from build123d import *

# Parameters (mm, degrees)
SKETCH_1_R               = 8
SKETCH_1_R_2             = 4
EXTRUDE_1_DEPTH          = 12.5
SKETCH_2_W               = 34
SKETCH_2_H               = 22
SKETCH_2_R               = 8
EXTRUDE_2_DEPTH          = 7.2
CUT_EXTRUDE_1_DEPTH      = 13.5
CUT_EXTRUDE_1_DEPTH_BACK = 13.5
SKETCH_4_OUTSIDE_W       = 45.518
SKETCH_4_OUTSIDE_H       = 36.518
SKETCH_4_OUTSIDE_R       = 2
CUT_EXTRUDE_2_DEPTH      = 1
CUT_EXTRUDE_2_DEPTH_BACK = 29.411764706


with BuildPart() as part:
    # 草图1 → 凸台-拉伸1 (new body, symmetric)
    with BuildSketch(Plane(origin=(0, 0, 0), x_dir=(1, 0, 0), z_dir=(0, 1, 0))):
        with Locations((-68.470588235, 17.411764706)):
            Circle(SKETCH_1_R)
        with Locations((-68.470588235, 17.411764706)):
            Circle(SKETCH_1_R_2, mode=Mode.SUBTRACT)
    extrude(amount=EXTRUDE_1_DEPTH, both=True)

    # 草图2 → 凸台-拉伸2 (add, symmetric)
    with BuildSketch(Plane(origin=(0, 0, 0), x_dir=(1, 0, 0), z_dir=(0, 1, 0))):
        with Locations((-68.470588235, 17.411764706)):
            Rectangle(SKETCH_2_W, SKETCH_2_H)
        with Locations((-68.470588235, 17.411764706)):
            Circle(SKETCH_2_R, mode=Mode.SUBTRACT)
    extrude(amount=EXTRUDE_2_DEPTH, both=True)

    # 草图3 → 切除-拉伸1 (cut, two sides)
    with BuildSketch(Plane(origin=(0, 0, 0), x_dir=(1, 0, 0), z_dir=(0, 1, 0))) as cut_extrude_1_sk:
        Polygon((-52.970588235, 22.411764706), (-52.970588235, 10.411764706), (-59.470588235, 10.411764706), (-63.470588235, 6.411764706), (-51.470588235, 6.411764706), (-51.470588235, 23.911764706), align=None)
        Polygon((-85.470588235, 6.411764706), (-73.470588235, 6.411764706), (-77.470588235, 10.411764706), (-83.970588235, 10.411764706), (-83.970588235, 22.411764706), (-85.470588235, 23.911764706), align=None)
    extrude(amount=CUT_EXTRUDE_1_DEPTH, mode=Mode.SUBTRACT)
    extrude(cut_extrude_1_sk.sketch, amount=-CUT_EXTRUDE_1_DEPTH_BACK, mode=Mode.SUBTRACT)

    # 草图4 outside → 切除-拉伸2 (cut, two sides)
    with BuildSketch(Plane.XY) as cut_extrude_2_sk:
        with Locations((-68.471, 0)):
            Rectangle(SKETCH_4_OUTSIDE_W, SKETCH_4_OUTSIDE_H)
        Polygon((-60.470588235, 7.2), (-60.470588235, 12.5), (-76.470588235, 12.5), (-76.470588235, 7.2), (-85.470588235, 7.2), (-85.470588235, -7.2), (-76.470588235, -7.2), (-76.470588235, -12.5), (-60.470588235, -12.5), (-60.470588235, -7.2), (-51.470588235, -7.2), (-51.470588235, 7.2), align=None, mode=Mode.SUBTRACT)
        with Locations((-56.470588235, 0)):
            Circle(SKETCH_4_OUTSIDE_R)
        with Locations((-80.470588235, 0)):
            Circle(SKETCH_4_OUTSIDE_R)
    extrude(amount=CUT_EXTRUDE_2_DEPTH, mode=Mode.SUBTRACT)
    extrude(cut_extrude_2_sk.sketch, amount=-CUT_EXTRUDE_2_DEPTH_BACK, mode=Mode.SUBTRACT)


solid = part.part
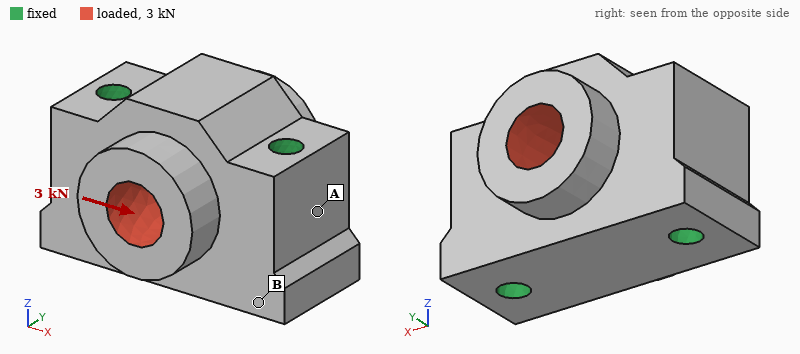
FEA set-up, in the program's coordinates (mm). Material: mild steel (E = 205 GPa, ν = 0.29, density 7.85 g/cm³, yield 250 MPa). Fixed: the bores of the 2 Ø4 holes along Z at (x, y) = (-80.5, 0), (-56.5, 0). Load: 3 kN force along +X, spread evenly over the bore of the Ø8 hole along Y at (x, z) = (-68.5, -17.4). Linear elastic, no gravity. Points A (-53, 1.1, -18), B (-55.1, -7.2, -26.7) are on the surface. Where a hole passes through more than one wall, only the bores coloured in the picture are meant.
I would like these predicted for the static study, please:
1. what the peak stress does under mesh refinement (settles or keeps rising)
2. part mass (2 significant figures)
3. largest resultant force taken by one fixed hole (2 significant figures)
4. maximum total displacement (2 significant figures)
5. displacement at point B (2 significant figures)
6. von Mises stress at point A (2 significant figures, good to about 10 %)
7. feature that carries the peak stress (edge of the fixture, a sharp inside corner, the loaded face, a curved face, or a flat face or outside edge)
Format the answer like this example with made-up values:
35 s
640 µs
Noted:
keeps rising
75 g
1.5 kN
0.82 µm
0.14 µm
5.3 MPa
edge of the fixture
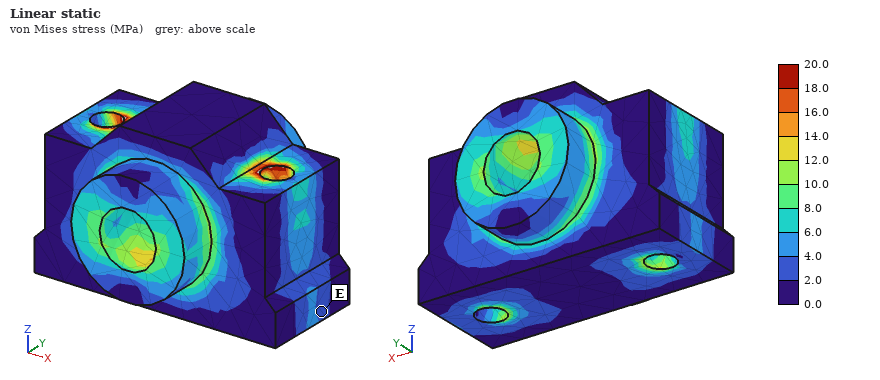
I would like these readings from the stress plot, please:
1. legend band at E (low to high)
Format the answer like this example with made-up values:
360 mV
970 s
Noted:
2.0 to 4.0 MPa
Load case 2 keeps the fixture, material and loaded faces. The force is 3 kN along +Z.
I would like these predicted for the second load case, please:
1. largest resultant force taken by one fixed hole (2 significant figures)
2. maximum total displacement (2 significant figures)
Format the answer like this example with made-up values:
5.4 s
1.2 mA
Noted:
1.5 kN
1.3 µm
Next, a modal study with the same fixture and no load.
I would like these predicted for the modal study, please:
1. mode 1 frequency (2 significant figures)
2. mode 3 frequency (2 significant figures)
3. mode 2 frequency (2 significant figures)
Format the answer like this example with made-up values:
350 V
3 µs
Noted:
37 kHz
48 kHz
48 kHz
